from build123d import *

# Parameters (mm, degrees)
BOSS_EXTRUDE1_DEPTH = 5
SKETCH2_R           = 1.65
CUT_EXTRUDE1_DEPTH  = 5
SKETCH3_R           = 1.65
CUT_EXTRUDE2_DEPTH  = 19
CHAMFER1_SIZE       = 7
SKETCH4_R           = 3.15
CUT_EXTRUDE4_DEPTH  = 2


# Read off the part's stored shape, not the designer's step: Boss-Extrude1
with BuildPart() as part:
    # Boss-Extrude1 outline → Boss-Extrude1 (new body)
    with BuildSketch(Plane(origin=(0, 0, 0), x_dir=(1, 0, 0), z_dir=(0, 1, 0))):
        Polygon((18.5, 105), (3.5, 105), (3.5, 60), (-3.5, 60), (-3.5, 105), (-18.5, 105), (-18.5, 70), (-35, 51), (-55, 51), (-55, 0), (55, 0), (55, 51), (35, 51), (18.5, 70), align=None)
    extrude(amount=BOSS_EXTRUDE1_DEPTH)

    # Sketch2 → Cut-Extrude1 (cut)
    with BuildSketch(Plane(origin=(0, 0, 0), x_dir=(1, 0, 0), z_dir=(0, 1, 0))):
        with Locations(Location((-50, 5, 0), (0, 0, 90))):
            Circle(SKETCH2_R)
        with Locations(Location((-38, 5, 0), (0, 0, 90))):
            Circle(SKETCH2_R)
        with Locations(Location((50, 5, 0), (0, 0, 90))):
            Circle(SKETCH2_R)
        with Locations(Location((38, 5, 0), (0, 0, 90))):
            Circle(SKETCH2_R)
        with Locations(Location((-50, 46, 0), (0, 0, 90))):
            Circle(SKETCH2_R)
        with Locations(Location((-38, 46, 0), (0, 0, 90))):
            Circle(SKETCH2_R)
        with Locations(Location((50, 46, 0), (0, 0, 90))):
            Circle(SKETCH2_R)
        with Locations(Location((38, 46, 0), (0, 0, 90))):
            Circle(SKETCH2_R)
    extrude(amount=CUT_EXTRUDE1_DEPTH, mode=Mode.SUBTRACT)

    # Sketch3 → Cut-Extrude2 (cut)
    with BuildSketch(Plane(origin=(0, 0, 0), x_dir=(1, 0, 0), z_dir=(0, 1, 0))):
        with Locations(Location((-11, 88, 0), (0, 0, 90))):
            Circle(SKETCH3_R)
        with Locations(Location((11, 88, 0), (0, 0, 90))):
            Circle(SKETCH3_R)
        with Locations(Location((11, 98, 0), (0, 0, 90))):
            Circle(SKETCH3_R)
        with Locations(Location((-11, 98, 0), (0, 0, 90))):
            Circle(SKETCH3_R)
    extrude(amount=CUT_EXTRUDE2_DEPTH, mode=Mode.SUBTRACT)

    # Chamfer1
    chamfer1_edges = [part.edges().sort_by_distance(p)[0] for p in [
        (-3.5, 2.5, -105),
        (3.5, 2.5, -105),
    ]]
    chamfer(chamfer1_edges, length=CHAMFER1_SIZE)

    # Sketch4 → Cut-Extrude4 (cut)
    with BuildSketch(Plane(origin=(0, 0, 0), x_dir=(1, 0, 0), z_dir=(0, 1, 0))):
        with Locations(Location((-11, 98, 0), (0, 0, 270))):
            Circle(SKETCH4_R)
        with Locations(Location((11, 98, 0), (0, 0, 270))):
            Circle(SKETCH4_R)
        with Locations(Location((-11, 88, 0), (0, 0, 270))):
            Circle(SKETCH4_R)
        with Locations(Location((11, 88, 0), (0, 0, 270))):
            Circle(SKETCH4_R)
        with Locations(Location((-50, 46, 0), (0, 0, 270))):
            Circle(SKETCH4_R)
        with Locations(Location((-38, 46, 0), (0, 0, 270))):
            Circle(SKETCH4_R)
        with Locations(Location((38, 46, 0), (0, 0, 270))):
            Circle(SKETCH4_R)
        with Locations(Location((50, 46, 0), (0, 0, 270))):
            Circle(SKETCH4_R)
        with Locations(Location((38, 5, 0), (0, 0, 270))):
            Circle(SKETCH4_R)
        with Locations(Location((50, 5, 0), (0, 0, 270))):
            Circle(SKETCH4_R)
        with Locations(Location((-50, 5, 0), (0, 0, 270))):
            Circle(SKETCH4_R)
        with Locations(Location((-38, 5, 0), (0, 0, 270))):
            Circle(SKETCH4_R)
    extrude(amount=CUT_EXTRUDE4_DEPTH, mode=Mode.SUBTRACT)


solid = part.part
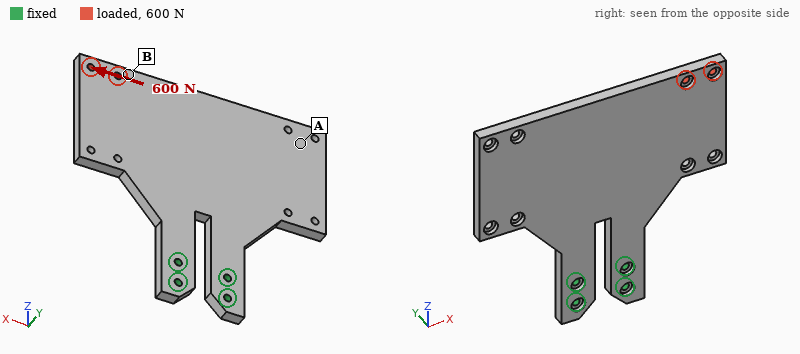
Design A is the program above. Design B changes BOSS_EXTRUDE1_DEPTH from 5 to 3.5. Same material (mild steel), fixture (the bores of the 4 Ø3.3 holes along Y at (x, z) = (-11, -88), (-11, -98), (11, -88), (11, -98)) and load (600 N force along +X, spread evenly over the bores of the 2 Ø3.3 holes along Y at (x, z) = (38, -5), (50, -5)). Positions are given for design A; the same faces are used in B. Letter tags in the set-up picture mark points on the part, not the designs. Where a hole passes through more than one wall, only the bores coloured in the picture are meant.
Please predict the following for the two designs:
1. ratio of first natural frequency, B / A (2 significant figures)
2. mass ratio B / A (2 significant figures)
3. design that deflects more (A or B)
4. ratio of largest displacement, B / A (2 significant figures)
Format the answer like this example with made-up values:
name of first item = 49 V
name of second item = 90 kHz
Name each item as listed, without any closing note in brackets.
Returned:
ratio of first natural frequency, B / A = 0.70
mass ratio B / A = 0.70
design that deflects more = B
ratio of largest displacement, B / A = 1.9
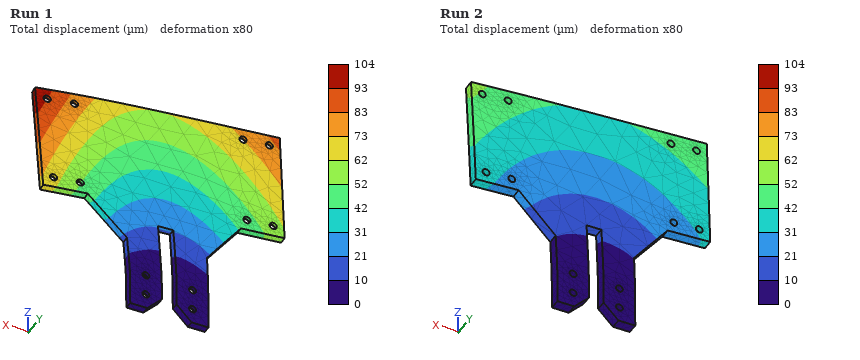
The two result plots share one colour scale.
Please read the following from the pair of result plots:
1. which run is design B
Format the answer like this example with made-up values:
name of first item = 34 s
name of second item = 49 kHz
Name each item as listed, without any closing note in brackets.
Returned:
which run is design B = Run 1
